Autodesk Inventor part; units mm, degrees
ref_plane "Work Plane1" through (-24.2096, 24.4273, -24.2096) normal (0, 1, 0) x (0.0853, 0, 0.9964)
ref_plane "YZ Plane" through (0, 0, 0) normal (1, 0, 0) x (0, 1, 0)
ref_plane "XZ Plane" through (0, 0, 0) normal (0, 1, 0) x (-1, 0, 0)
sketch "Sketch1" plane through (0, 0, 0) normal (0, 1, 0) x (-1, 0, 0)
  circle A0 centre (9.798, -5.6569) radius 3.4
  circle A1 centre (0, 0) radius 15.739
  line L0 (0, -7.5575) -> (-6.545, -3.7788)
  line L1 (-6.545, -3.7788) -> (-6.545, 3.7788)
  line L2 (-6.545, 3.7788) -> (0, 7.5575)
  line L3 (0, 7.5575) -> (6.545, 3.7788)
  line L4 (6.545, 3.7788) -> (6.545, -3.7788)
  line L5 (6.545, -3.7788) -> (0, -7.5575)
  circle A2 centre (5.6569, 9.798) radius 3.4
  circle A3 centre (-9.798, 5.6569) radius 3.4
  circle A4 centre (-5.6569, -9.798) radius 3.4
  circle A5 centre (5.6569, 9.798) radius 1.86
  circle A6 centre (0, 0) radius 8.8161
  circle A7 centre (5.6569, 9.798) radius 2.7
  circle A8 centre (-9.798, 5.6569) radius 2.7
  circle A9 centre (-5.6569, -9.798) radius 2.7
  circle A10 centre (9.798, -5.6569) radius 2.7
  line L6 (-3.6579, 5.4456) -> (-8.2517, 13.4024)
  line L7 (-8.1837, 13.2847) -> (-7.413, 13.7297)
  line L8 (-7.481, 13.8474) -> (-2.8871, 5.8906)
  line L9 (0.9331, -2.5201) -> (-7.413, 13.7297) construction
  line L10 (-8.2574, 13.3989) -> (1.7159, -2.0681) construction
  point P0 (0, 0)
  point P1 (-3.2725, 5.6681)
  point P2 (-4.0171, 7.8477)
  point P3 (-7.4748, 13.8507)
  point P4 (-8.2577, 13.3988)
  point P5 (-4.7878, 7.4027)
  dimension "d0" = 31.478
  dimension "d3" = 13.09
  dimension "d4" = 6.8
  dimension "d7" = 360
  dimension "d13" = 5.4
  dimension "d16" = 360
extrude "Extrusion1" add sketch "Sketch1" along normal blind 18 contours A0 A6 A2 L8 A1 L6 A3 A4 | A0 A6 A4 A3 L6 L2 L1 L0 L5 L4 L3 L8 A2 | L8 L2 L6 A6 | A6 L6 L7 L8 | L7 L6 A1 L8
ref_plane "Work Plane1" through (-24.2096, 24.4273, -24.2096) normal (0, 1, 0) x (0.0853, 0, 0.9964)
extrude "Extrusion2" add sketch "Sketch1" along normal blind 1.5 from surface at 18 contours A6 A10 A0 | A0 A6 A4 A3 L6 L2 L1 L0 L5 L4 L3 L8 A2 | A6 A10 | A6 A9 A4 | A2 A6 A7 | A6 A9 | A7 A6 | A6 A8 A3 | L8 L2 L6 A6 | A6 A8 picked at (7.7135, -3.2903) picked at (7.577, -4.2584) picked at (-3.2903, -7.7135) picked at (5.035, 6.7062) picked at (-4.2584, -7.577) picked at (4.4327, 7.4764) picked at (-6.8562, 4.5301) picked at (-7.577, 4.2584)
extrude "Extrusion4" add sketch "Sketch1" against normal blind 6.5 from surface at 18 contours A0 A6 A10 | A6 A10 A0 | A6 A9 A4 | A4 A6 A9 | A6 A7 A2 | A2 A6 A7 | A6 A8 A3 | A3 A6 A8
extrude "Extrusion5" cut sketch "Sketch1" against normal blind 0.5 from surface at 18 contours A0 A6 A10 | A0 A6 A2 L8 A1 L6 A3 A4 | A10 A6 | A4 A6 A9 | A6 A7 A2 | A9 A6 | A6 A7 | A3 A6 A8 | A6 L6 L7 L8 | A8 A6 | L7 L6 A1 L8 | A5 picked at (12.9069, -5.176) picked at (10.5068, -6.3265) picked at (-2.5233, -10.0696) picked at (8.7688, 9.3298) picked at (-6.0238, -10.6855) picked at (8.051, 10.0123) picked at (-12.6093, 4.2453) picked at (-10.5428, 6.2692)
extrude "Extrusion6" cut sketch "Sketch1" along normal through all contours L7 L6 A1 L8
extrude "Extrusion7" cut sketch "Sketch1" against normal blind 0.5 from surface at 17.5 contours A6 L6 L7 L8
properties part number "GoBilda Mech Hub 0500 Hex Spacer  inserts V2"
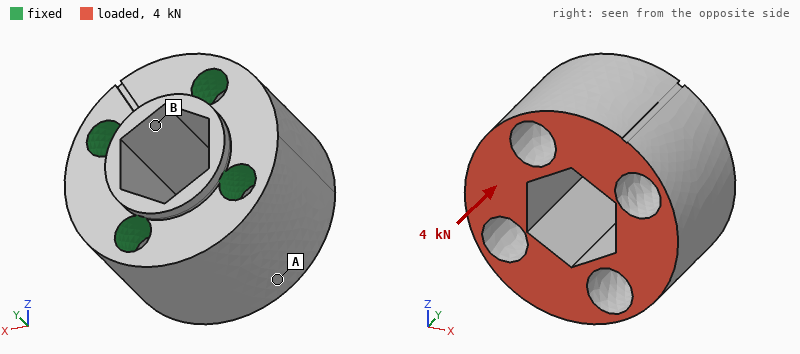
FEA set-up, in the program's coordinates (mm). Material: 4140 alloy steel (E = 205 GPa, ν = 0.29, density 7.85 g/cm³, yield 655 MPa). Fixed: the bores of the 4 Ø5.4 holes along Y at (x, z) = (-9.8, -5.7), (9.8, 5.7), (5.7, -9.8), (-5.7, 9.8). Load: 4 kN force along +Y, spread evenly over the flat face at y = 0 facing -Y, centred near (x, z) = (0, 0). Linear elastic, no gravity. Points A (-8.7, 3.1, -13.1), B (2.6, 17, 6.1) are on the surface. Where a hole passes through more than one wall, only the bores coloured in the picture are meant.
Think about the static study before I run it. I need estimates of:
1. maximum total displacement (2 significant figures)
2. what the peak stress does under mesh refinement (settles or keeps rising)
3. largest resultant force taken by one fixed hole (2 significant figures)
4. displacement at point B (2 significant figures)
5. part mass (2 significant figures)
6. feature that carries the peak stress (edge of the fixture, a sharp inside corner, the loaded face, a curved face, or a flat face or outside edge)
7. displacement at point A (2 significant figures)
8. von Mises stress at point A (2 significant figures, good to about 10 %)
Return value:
0.96 µm
keeps rising
1.0 kN
0.22 µm
71 g
edge of the fixture
0.79 µm
8.5 MPa
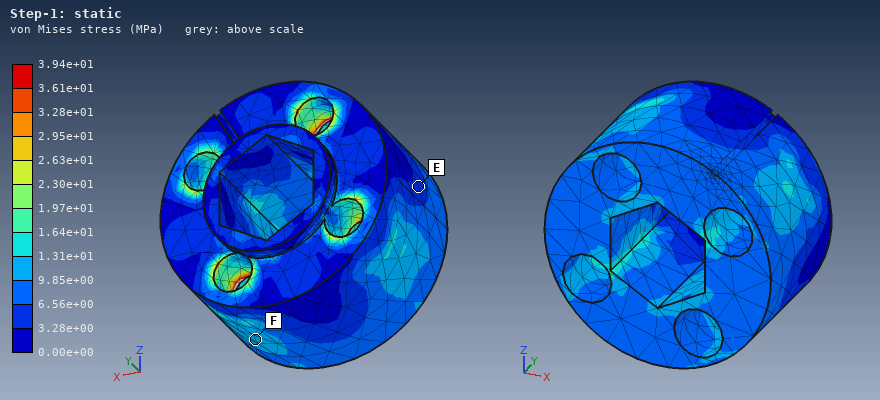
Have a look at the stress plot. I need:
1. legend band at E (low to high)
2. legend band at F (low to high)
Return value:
3.28e+00 to 6.56e+00 MPa
9.85e+00 to 1.31e+01 MPa
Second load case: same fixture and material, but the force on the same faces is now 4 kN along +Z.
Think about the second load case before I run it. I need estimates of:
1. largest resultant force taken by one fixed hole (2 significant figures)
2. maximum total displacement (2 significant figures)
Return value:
1.8 kN
6.3 µm
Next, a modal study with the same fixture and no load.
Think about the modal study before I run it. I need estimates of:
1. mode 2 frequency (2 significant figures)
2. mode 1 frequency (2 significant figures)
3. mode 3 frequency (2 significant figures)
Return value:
32 kHz
30 kHz
33 kHz
